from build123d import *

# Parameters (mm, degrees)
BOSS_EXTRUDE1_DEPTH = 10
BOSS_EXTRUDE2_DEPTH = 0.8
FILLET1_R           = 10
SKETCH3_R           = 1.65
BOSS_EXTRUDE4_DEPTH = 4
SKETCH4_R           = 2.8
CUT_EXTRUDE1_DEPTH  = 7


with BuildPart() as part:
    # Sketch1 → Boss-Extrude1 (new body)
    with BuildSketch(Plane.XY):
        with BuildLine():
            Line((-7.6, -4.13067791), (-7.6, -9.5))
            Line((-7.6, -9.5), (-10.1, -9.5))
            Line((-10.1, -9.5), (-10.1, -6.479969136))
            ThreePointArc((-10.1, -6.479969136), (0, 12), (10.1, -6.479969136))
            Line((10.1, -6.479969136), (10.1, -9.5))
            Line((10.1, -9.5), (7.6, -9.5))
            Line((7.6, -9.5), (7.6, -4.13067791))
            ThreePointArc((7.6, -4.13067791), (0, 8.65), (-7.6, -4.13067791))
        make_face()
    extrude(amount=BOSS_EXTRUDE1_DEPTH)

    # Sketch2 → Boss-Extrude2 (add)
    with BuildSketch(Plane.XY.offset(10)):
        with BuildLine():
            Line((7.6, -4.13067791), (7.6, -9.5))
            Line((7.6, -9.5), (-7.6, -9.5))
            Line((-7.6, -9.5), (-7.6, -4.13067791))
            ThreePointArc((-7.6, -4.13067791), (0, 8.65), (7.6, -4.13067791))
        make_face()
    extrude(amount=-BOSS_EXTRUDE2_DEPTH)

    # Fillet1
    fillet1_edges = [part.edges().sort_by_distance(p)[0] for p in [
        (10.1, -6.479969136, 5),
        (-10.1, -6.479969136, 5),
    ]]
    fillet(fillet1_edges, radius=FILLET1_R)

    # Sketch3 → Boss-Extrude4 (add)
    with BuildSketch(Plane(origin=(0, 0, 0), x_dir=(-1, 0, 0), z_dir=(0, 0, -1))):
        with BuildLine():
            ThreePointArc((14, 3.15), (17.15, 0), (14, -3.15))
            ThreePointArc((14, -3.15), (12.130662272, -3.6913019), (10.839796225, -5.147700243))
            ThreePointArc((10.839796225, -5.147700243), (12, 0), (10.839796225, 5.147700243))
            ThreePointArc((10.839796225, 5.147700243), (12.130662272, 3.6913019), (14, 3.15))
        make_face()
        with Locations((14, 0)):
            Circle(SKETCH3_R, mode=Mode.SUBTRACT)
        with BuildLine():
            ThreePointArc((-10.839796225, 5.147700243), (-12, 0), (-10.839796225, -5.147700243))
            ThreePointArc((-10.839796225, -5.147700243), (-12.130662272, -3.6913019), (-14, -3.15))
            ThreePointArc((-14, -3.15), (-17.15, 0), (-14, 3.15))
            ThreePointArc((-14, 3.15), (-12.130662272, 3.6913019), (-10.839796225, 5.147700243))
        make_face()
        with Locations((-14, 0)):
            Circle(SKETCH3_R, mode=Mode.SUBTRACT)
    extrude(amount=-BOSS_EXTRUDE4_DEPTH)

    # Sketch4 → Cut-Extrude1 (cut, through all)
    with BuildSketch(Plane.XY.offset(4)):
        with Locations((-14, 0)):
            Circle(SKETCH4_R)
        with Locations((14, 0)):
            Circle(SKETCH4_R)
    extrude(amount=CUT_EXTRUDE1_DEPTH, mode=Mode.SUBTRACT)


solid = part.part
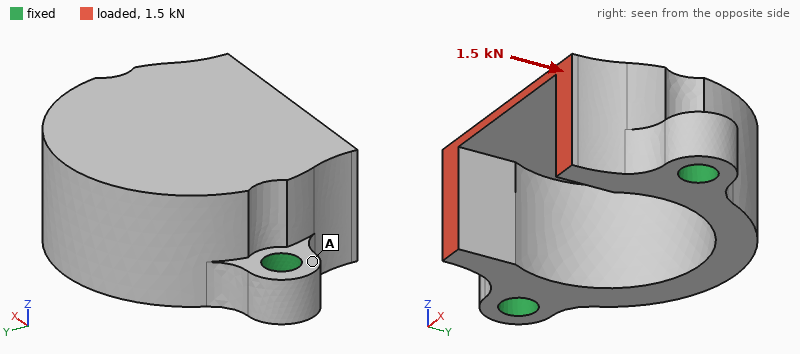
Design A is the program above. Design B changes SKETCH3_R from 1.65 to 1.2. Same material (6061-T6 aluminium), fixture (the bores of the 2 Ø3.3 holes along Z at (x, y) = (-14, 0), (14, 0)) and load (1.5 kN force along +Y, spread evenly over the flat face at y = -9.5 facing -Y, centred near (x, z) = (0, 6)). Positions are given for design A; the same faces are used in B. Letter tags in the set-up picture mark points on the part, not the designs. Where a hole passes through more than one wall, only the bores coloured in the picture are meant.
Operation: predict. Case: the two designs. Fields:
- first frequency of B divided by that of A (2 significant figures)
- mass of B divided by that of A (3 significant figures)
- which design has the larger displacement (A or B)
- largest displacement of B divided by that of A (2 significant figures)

0.89
1.02
B
1.3
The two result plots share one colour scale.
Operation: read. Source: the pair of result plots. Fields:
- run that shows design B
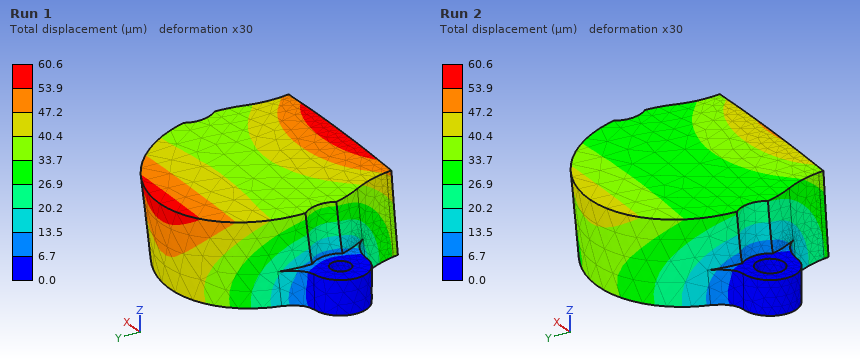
Run 1
